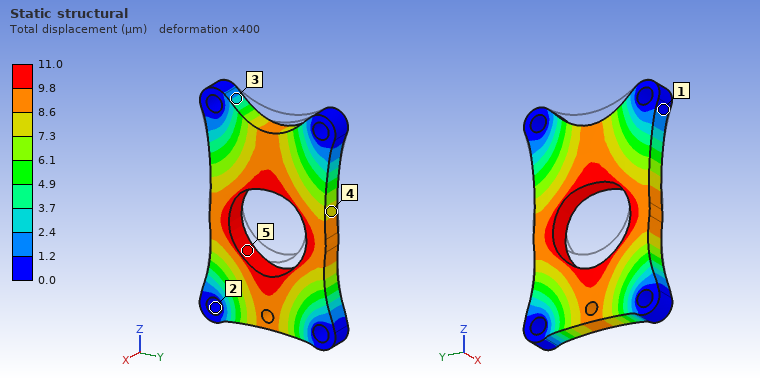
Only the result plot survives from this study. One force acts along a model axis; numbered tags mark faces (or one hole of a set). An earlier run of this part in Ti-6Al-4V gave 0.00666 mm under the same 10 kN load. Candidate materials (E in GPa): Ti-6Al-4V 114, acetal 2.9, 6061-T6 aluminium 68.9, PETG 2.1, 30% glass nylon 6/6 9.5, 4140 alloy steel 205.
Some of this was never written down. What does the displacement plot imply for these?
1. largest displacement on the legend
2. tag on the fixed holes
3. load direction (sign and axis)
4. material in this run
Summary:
11.0 µm
2
-Z
6061-T6 aluminium
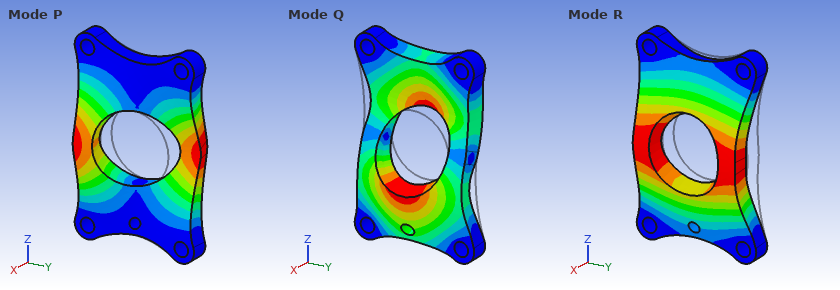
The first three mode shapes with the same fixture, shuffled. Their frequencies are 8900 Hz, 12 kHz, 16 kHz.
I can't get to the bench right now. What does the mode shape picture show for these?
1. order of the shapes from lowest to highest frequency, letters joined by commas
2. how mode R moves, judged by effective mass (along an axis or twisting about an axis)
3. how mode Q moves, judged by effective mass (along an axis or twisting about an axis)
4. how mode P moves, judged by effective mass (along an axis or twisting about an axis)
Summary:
R, P, Q
along X
twisting about Y
twisting about Z
